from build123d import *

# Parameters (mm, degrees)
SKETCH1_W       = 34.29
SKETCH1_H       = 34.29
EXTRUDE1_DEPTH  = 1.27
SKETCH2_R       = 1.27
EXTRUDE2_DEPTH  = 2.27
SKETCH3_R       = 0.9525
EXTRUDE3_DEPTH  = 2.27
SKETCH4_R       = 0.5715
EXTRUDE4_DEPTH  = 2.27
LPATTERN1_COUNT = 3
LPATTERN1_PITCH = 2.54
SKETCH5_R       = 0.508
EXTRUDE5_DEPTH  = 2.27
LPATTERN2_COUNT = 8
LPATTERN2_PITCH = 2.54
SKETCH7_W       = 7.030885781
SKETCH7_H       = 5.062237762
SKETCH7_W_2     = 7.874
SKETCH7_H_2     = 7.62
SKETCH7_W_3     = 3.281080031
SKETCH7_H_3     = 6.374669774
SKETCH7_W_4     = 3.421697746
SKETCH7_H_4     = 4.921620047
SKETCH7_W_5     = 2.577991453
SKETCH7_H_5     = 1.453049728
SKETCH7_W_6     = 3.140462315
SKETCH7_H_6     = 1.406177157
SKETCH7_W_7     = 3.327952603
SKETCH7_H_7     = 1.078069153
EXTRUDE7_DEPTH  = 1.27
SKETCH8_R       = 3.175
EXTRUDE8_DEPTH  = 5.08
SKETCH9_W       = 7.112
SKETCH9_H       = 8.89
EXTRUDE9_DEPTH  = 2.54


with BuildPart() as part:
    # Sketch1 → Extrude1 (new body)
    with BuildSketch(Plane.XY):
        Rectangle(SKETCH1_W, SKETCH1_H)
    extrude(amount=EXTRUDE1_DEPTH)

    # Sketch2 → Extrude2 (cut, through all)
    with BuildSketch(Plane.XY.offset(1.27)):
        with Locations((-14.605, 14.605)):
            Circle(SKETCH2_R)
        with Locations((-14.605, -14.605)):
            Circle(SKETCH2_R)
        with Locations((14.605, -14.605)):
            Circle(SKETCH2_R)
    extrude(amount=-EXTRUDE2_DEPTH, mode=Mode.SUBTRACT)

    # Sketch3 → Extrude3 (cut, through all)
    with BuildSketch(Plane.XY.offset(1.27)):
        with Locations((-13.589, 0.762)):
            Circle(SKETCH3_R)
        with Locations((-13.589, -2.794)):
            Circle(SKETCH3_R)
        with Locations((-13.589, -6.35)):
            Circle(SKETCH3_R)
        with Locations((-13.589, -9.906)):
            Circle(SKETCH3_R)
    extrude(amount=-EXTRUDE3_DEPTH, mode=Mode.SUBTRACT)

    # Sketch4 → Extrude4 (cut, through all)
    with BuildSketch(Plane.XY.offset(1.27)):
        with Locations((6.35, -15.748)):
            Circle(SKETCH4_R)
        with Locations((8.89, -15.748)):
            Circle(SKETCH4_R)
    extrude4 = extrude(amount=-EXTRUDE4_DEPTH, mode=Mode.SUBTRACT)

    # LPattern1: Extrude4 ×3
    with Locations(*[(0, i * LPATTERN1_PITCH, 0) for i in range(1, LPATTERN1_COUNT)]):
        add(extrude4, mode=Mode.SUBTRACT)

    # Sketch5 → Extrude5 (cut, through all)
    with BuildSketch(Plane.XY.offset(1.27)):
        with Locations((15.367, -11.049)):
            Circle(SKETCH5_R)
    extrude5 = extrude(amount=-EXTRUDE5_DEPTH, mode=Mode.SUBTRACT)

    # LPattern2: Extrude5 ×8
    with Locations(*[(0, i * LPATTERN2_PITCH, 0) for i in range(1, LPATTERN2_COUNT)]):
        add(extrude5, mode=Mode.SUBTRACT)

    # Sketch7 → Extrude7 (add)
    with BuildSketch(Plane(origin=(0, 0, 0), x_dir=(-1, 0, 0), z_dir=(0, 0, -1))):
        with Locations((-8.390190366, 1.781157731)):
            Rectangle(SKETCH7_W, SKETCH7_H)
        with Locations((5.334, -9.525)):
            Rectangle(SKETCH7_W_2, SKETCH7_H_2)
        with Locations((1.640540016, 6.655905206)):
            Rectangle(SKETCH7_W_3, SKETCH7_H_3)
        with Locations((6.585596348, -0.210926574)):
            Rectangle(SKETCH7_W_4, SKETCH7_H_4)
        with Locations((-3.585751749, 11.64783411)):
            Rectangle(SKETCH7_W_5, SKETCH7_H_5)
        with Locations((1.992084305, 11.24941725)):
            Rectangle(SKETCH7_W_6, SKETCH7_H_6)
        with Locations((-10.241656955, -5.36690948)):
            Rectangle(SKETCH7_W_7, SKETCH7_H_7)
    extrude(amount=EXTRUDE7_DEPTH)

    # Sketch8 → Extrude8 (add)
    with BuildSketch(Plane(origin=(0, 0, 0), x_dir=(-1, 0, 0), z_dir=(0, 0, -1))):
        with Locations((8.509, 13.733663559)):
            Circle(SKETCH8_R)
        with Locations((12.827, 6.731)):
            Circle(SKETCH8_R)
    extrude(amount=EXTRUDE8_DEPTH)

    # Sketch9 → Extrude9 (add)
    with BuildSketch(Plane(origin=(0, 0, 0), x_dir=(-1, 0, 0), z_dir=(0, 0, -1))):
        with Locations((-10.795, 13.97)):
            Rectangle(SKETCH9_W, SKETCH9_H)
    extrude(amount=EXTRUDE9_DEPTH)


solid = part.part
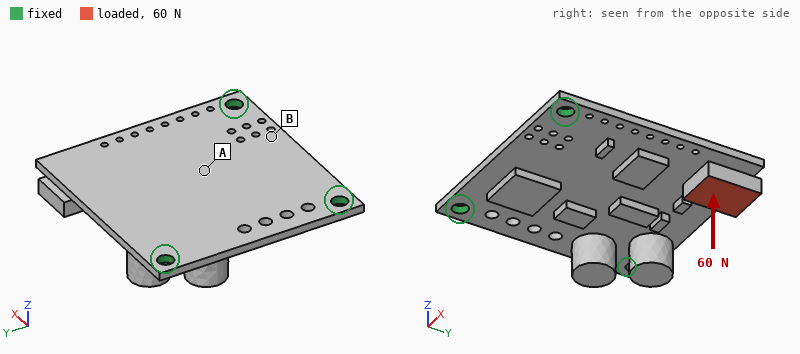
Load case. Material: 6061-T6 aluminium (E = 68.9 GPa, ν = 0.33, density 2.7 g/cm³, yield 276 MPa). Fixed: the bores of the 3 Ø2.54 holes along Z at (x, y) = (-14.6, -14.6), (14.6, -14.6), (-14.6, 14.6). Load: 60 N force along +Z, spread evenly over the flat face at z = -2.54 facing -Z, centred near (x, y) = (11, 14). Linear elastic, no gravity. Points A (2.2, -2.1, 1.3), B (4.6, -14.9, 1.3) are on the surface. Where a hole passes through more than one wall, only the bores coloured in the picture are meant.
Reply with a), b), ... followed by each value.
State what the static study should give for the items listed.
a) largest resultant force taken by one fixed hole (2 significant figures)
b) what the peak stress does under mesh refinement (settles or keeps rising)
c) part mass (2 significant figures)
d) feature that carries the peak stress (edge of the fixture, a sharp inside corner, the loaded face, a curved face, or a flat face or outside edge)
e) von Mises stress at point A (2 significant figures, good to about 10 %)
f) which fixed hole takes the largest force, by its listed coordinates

a) 51 N
b) keeps rising
c) 5.7 g
d) edge of the fixture
e) 46 MPa
f) (-14.6, 14.6)
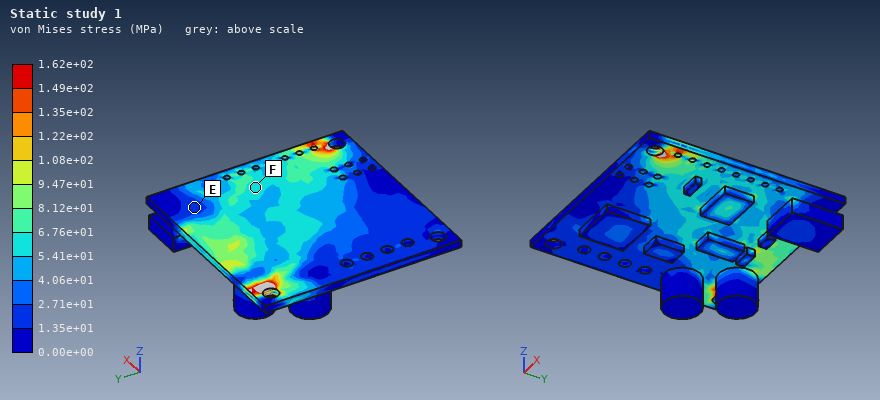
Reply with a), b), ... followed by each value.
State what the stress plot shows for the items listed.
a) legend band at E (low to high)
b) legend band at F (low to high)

a) 1.35e+01 to 2.71e+01 MPa
b) 5.41e+01 to 6.76e+01 MPa
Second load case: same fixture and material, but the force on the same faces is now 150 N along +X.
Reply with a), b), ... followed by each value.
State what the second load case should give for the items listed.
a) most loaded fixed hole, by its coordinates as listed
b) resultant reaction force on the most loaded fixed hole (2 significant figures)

a) (-14.6, 14.6)
b) 100 N
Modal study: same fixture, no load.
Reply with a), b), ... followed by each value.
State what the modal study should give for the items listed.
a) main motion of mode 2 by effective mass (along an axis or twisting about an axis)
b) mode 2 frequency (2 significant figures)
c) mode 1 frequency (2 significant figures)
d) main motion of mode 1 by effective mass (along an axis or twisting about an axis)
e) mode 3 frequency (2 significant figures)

a) along Z
b) 5100 Hz
c) 1800 Hz
d) along Z
e) 7000 Hz
